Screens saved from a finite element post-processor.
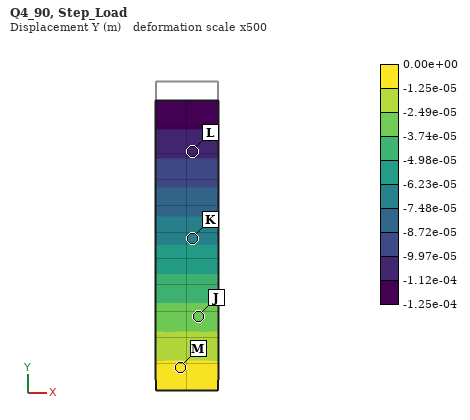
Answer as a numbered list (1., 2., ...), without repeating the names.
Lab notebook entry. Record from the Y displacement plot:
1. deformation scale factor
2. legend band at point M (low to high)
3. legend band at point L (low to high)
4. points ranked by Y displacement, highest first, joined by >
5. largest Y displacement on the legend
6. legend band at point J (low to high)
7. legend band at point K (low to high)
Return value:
1. 500
2. -1.25e-05 to 0.00e+00 m
3. -1.12e-04 to -9.97e-05 m
4. M > J > K > L
5. 0.00e+00 m
6. -3.74e-05 to -2.49e-05 m
7. -7.48e-05 to -6.23e-05 m
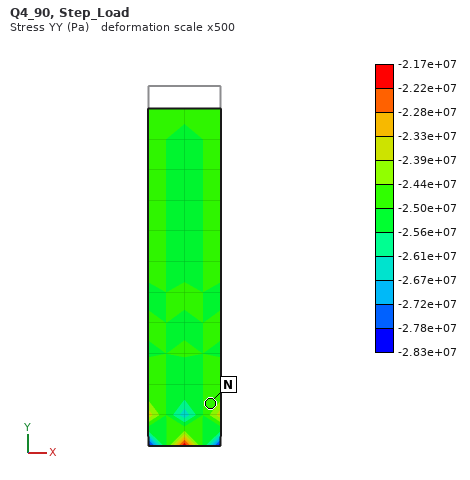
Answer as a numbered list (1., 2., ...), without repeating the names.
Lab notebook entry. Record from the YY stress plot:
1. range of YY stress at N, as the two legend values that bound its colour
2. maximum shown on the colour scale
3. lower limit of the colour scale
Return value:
1. -2.50e+07 to -2.44e+07 Pa
2. -2.17e+07 Pa
3. -2.83e+07 Pa
